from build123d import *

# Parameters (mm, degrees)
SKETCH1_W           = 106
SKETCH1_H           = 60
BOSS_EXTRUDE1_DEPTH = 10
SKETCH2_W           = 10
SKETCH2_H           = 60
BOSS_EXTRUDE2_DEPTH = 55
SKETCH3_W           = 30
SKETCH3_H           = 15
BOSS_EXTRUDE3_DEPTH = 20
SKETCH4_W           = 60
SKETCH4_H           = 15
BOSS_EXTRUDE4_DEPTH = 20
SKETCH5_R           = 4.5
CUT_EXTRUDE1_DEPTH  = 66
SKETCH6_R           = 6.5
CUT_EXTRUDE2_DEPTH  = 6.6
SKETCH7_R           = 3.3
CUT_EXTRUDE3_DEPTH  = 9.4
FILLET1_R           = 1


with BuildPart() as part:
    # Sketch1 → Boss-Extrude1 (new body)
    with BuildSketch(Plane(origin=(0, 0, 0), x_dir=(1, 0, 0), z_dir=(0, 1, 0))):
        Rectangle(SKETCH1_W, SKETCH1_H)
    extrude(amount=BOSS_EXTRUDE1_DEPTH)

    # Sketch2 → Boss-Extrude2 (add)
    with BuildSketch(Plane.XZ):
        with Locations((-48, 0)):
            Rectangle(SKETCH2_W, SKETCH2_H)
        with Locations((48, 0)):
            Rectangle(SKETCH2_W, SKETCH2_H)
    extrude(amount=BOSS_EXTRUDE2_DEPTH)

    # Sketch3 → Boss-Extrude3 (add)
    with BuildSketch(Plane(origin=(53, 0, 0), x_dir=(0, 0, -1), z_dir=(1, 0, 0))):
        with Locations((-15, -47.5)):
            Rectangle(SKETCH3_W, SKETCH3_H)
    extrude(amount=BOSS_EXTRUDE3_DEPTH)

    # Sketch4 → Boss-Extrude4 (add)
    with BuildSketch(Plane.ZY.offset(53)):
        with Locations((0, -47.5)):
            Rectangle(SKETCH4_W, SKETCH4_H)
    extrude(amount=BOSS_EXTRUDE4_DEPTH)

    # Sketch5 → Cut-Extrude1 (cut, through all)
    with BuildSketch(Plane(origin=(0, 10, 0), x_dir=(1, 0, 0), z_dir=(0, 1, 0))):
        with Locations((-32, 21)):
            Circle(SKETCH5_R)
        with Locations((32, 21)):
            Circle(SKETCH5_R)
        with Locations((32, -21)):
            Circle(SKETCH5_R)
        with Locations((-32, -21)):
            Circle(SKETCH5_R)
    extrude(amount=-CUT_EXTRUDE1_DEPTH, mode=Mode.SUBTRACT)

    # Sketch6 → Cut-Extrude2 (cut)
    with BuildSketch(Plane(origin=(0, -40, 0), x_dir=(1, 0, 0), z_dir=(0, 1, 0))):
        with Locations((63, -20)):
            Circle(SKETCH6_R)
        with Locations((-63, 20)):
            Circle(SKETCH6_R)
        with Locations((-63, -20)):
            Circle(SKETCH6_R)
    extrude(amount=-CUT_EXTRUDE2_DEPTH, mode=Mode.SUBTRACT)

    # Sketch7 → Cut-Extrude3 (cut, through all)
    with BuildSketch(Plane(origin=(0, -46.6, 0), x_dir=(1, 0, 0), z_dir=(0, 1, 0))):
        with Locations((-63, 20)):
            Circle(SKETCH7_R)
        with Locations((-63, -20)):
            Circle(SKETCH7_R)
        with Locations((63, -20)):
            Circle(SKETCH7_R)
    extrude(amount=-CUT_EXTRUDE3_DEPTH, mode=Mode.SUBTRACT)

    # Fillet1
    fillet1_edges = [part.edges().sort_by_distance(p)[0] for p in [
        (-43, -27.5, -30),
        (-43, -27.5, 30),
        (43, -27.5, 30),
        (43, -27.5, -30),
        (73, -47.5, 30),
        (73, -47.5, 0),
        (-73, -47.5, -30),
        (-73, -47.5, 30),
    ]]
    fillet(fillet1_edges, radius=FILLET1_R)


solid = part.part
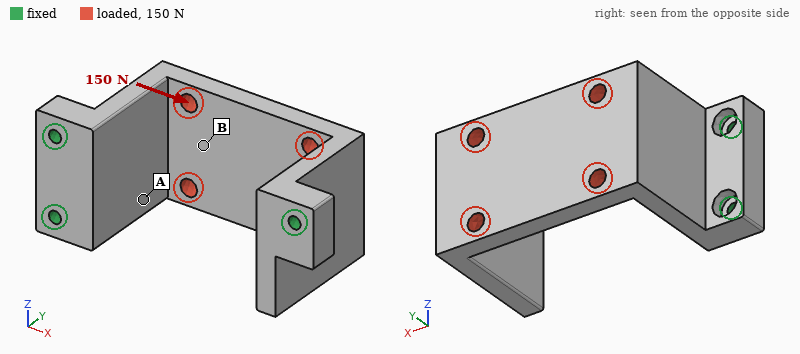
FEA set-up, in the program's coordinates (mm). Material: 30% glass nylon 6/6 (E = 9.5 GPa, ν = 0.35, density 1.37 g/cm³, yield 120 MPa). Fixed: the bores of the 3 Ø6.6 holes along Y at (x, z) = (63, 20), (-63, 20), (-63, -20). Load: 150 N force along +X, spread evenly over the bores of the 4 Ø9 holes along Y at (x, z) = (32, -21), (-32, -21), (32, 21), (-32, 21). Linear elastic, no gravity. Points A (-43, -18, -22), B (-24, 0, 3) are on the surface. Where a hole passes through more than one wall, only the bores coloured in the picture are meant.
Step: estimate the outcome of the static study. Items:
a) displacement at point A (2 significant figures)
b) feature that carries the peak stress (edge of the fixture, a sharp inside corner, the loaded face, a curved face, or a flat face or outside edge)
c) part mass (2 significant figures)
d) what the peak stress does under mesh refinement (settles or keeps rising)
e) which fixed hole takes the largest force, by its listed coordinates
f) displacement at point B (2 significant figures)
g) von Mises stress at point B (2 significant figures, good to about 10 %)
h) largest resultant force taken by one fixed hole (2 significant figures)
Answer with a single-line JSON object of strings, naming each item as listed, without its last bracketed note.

{"displacement at point A": "27 µm", "feature that carries the peak stress": "edge of the fixture", "part mass": "210 g", "what the peak stress does under mesh refinement": "keeps rising", "which fixed hole takes the largest force, by its listed coordinates": "(63, 20)", "displacement at point B": "48 µm", "von Mises stress at point B": "1.2 MPa", "largest resultant force taken by one fixed hole": "77 N"}
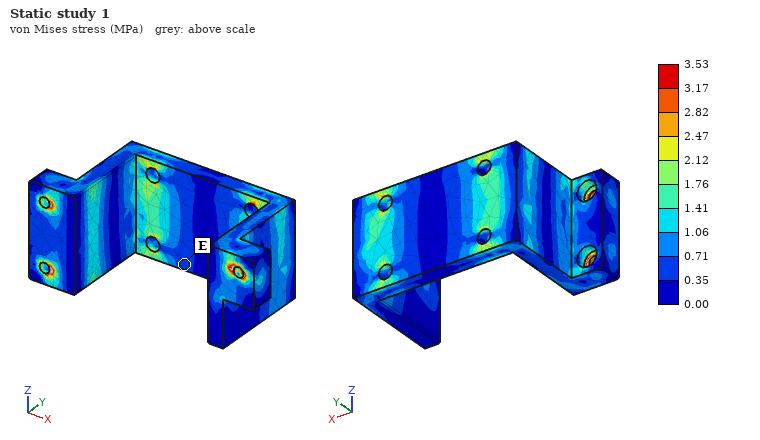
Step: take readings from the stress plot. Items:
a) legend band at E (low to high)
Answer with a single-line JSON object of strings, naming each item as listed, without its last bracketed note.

{"legend band at E": "0.35 to 0.71 MPa"}
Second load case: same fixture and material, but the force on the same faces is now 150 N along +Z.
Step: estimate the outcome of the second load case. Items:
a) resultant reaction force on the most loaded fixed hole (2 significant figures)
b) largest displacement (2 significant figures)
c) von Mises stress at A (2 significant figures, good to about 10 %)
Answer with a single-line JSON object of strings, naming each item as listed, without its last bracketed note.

{"resultant reaction force on the most loaded fixed hole": "160 N", "largest displacement": "79 µm", "von Mises stress at A": "1.1 MPa"}
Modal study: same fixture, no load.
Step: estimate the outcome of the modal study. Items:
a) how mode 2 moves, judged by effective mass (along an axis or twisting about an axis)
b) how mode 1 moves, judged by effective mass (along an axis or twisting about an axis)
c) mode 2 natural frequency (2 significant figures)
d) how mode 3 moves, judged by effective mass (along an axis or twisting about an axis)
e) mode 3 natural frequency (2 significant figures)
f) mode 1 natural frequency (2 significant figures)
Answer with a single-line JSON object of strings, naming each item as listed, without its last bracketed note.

{"how mode 2 moves, judged by effective mass": "along X", "how mode 1 moves, judged by effective mass": "along Z", "mode 2 natural frequency": "850 Hz", "how mode 3 moves, judged by effective mass": "along Z", "mode 3 natural frequency": "1900 Hz", "mode 1 natural frequency": "760 Hz"}
